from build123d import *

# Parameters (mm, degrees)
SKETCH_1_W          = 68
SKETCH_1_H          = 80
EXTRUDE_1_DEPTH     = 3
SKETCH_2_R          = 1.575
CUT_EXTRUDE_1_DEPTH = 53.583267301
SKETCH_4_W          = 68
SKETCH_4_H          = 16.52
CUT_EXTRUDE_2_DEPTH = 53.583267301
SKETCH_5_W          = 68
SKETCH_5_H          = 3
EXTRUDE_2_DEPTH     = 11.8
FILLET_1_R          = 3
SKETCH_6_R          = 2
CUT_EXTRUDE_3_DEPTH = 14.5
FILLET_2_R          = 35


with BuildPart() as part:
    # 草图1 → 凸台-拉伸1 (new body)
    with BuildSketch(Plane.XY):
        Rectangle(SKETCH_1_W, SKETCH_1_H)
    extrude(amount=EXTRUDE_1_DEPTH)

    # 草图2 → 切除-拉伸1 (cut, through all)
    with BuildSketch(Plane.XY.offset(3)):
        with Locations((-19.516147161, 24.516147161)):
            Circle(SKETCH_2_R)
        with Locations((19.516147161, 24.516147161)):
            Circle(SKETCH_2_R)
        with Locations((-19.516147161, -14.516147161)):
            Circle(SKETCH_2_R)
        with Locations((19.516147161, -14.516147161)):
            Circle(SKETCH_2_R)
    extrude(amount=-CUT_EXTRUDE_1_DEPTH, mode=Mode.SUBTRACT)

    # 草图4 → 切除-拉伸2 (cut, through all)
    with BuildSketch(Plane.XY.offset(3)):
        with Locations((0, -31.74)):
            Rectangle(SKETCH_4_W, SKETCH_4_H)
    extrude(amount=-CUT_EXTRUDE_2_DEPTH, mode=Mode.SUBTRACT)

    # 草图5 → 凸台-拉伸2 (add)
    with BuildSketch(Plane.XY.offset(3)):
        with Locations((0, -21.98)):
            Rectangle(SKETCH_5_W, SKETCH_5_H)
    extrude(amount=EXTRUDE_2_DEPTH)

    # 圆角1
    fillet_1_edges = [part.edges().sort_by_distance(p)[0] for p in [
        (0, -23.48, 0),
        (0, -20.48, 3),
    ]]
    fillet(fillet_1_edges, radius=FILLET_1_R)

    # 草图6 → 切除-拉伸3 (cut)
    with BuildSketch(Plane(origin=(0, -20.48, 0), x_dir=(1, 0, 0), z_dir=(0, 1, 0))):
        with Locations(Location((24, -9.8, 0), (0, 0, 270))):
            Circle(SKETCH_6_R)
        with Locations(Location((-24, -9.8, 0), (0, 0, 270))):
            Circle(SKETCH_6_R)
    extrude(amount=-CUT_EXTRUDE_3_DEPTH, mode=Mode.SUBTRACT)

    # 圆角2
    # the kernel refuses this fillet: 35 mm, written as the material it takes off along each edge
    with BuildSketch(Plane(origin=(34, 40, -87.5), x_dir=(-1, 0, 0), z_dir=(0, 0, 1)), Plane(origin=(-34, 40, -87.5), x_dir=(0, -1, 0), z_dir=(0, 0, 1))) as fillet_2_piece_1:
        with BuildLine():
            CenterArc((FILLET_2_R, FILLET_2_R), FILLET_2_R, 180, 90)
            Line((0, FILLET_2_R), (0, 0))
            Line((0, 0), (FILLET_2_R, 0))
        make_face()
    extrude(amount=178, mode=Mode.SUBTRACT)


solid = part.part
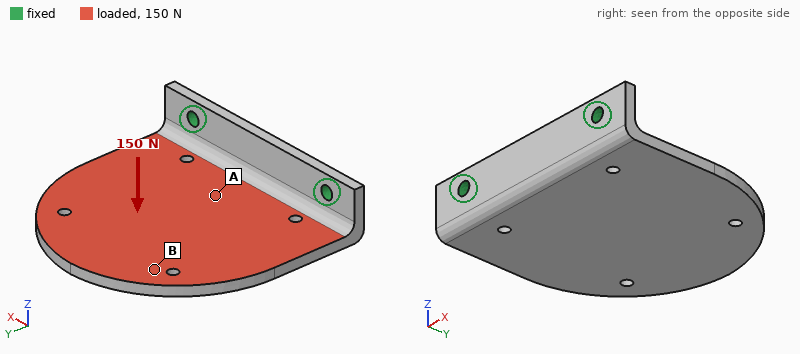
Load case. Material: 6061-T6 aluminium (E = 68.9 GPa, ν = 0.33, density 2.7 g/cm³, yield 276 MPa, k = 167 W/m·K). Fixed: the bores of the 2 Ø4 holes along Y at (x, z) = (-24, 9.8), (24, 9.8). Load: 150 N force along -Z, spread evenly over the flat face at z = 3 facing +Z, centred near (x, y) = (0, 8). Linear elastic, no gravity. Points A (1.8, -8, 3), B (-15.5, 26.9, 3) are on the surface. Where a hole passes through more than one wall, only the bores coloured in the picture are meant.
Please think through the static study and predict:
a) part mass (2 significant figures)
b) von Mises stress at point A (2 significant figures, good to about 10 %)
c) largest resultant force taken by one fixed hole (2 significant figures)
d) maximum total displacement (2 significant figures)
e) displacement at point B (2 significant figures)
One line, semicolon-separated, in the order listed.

37 g; 23 MPa; 85 N; 0.59 mm; 0.44 mm
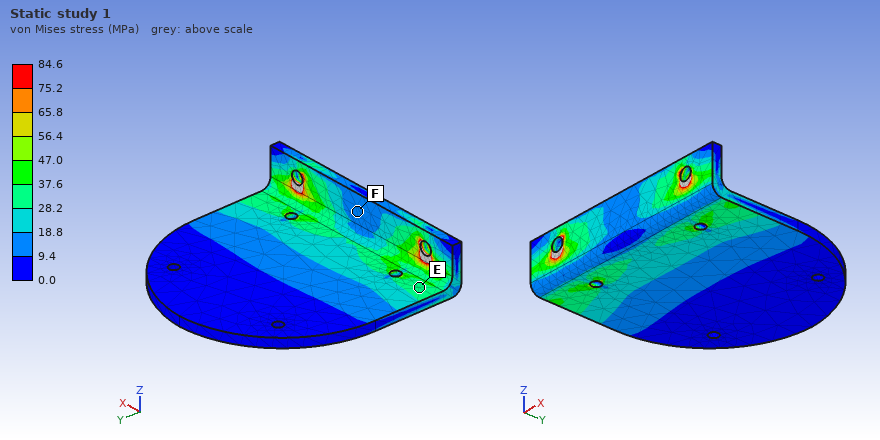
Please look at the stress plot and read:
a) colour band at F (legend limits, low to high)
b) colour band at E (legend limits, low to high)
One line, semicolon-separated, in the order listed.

9.4 to 18.8 MPa; 28.2 to 37.6 MPa
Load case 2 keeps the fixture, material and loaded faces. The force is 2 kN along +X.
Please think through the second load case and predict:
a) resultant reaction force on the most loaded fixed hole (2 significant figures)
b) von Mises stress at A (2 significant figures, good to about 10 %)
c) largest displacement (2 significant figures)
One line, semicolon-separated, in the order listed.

1.6 kN; 49 MPa; 0.29 mm
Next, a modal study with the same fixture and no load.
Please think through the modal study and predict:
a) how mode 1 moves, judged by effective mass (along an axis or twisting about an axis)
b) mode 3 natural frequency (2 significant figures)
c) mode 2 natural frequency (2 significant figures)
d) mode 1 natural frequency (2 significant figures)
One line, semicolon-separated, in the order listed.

along Z; 3500 Hz; 1900 Hz; 640 Hz
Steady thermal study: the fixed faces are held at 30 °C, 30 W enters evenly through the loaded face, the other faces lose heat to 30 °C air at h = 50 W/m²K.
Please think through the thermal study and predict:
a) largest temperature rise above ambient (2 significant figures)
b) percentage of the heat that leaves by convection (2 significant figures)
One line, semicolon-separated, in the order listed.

32 K; 20 %
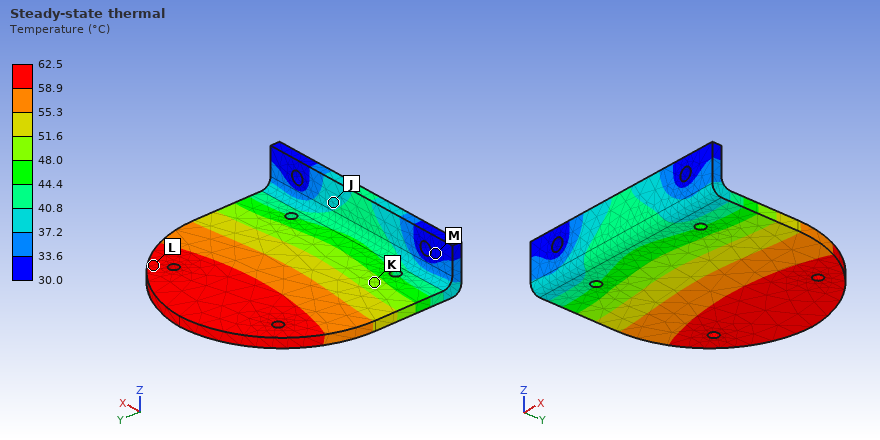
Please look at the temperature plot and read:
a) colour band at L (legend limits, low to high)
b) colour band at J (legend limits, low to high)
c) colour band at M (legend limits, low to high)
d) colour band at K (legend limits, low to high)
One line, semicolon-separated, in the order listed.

58.9 to 62.5 °C; 37.2 to 40.8 °C; 30.0 to 33.6 °C; 48.0 to 51.6 °C
